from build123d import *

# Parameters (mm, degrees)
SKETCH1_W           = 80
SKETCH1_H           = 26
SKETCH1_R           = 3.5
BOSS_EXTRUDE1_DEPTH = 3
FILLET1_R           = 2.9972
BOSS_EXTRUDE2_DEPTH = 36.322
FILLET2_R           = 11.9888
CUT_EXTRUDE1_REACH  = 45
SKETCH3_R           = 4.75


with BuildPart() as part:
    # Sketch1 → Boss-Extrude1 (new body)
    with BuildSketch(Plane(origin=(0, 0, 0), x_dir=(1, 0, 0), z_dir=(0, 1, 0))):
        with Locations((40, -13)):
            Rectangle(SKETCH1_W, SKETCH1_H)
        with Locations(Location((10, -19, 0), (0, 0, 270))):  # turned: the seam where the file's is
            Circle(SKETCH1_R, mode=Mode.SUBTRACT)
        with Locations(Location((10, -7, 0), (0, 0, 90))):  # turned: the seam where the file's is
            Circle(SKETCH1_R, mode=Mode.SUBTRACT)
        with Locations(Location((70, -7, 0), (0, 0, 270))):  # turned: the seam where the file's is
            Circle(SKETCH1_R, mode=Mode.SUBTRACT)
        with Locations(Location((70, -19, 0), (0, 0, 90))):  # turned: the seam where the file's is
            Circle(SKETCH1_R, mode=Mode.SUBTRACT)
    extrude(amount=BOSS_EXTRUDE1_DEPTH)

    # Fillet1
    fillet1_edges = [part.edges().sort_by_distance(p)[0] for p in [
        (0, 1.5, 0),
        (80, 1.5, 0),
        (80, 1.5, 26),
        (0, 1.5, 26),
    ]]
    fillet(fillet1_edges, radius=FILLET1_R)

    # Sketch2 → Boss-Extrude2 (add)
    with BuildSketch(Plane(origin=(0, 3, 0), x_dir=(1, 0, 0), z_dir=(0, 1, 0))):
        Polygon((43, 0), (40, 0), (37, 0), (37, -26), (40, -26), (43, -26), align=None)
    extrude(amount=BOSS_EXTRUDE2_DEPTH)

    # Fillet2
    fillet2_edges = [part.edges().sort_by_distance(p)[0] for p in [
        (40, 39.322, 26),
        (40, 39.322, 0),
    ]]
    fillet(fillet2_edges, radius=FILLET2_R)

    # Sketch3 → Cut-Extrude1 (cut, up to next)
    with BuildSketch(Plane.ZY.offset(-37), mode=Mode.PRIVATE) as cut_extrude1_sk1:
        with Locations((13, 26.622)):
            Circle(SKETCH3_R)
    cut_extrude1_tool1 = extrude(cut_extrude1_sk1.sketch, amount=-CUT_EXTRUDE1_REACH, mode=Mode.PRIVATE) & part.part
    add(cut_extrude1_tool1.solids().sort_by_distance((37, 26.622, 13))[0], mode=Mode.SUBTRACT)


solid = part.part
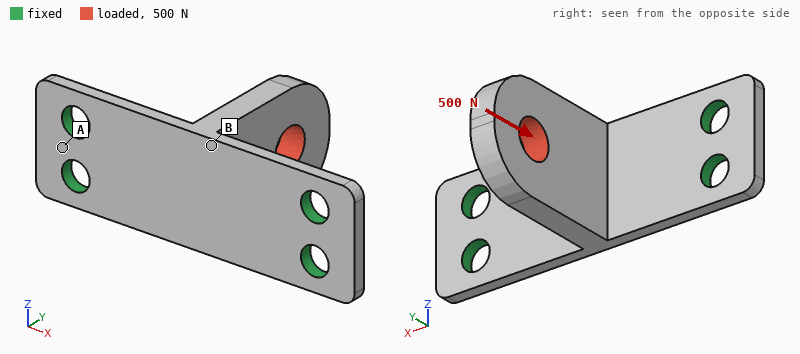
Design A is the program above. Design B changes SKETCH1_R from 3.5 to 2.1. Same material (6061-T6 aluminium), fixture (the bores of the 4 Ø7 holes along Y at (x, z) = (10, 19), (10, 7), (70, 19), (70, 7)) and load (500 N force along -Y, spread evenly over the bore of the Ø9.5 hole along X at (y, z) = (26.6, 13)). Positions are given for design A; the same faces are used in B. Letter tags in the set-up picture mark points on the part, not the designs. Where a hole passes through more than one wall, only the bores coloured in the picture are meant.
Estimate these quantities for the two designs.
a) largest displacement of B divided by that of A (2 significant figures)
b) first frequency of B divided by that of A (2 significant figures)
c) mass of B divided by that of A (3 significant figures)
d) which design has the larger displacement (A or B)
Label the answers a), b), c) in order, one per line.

a) 1.2
b) 0.94
c) 1.03
d) B
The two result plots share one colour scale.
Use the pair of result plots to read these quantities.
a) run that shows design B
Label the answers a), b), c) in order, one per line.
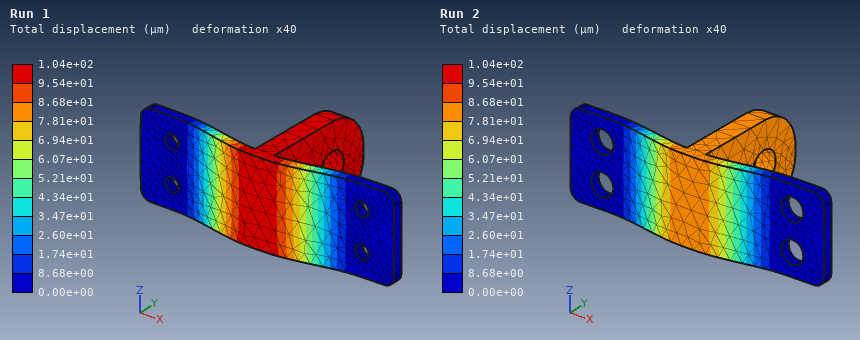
a) Run 1
